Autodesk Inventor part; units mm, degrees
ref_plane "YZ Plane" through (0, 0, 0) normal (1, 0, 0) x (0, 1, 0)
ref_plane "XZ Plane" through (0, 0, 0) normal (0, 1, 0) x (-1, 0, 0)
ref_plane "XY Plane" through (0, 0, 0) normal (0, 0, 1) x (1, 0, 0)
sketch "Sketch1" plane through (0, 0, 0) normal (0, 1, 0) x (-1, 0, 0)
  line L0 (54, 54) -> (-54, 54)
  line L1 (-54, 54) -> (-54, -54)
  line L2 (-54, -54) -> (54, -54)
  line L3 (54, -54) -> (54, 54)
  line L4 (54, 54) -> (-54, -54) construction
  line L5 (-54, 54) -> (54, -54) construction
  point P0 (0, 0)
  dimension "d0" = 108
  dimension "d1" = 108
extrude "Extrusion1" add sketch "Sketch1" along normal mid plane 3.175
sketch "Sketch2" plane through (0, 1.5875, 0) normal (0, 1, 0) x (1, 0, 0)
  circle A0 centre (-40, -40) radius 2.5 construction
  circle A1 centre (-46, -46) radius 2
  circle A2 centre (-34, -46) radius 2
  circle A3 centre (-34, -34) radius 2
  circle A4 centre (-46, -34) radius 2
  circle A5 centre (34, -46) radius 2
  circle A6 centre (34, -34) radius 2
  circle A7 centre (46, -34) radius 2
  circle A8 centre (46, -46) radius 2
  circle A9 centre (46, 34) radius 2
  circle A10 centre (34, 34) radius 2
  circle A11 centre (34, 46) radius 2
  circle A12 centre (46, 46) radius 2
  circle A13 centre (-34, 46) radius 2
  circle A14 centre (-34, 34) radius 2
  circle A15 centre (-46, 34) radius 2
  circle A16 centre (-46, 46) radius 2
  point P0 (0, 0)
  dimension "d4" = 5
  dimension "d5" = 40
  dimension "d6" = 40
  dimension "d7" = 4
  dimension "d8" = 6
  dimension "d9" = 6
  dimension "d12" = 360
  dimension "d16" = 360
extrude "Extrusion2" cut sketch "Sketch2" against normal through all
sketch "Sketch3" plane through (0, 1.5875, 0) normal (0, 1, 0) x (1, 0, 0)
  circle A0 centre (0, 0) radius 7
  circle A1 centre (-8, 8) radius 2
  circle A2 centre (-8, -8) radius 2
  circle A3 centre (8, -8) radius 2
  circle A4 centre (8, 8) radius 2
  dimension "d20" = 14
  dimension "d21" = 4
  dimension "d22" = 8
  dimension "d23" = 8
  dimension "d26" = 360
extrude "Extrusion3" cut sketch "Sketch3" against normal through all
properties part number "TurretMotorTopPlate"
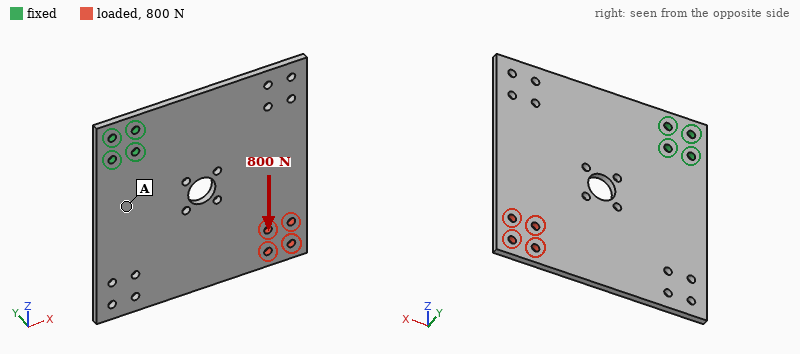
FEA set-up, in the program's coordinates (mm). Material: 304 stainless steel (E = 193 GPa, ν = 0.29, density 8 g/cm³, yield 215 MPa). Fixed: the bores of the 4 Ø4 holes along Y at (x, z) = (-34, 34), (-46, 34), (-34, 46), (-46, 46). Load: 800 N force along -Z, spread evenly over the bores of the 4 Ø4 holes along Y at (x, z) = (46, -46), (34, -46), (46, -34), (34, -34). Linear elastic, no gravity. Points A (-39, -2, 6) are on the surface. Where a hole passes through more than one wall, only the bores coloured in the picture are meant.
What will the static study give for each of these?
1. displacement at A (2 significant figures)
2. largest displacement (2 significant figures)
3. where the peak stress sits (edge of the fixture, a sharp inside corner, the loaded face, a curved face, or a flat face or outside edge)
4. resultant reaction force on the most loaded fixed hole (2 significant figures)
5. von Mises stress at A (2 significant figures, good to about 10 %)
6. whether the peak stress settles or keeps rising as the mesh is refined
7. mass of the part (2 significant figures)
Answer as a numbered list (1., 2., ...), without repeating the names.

1. 14 µm
2. 67 µm
3. edge of the fixture
4. 2.2 kN
5. 11 MPa
6. keeps rising
7. 290 g
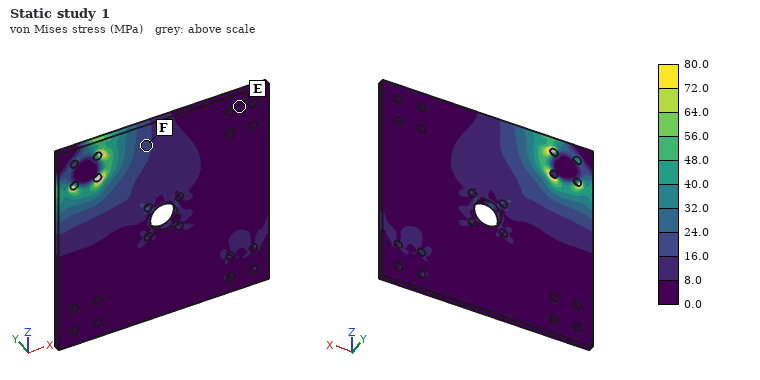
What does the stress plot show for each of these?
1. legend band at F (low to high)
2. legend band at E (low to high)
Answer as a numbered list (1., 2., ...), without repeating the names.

1. 16.0 to 24.0 MPa
2. 0.0 to 8.0 MPa
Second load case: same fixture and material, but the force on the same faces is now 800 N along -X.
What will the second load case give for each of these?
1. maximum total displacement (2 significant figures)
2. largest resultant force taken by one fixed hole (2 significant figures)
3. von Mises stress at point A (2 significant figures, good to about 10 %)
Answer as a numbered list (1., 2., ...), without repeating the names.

1. 67 µm
2. 2.2 kN
3. 15 MPa
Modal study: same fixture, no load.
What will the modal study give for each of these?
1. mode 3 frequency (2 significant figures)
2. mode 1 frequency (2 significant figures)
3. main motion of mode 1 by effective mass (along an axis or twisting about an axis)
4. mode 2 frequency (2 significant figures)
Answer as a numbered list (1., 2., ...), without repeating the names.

1. 770 Hz
2. 190 Hz
3. along Y
4. 350 Hz
